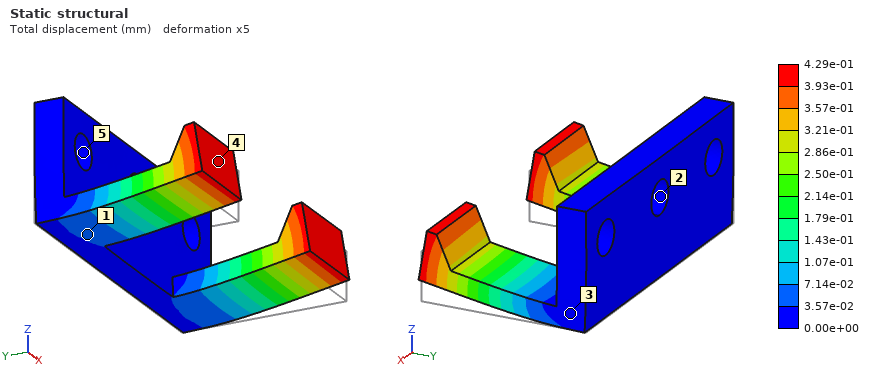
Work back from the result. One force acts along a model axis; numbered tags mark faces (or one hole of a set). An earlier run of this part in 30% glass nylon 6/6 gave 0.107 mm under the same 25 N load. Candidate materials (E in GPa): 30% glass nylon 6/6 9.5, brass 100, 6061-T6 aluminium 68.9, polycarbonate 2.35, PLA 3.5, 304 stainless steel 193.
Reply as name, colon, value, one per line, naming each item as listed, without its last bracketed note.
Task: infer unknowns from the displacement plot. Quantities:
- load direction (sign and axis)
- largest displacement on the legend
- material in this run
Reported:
load direction: +Z
largest displacement on the legend: 4.29e-01 mm
material in this run: polycarbonate
